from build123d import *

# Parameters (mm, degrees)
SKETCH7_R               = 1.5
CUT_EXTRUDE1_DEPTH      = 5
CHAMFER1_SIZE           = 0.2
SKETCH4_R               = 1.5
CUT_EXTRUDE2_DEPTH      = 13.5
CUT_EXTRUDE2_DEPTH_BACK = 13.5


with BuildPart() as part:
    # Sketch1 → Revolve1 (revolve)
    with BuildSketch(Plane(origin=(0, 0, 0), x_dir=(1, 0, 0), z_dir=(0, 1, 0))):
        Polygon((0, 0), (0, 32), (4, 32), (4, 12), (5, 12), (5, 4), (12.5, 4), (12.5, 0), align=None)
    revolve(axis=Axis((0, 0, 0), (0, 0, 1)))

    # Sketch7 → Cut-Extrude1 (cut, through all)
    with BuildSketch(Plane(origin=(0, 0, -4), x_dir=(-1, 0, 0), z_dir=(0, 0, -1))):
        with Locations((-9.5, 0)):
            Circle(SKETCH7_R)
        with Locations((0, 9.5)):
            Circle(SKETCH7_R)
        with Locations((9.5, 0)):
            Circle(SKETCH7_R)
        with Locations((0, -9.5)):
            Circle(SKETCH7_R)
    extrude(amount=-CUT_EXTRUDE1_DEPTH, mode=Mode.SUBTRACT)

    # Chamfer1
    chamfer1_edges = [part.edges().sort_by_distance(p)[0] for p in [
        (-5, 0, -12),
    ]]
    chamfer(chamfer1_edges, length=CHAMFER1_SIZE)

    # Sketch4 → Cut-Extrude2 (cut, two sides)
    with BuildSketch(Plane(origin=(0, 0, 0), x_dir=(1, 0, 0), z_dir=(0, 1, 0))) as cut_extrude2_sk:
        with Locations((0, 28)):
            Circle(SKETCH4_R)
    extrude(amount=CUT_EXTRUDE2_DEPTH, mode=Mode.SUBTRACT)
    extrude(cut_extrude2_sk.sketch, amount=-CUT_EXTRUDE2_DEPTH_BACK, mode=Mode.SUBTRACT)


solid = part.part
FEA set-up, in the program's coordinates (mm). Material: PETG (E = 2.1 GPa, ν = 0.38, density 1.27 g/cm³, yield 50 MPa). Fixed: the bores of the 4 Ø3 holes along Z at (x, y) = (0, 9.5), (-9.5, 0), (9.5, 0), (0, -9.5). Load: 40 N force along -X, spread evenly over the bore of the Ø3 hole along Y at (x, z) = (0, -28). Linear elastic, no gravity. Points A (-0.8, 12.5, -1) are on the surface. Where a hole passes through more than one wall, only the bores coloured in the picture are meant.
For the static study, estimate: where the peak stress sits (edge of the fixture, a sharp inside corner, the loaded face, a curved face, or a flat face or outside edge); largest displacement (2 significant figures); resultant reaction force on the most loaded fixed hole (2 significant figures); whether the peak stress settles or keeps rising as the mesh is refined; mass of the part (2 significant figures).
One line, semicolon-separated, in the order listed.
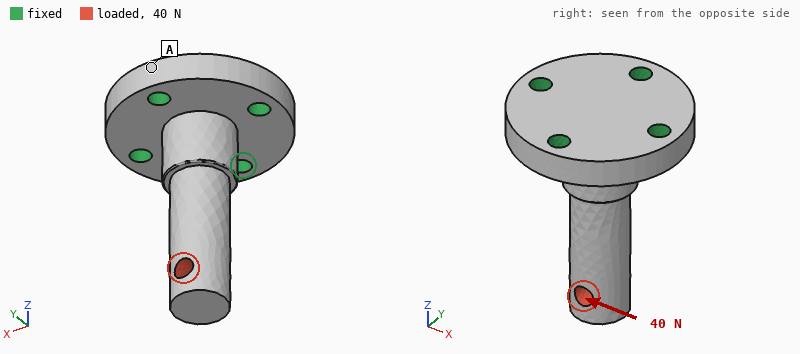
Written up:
a sharp inside corner; 0.48 mm; 63 N; keeps rising; 4.4 g
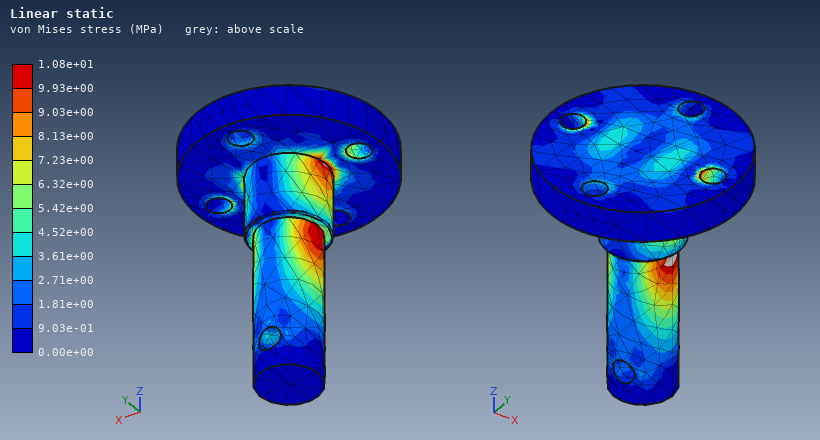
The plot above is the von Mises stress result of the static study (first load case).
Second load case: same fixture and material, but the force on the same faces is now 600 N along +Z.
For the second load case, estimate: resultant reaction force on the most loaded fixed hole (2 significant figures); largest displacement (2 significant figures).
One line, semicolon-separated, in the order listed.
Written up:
160 N; 0.21 mm
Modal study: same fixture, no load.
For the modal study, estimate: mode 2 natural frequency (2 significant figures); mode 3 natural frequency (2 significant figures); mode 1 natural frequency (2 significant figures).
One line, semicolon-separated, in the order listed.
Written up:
2000 Hz; 8000 Hz; 2000 Hz
